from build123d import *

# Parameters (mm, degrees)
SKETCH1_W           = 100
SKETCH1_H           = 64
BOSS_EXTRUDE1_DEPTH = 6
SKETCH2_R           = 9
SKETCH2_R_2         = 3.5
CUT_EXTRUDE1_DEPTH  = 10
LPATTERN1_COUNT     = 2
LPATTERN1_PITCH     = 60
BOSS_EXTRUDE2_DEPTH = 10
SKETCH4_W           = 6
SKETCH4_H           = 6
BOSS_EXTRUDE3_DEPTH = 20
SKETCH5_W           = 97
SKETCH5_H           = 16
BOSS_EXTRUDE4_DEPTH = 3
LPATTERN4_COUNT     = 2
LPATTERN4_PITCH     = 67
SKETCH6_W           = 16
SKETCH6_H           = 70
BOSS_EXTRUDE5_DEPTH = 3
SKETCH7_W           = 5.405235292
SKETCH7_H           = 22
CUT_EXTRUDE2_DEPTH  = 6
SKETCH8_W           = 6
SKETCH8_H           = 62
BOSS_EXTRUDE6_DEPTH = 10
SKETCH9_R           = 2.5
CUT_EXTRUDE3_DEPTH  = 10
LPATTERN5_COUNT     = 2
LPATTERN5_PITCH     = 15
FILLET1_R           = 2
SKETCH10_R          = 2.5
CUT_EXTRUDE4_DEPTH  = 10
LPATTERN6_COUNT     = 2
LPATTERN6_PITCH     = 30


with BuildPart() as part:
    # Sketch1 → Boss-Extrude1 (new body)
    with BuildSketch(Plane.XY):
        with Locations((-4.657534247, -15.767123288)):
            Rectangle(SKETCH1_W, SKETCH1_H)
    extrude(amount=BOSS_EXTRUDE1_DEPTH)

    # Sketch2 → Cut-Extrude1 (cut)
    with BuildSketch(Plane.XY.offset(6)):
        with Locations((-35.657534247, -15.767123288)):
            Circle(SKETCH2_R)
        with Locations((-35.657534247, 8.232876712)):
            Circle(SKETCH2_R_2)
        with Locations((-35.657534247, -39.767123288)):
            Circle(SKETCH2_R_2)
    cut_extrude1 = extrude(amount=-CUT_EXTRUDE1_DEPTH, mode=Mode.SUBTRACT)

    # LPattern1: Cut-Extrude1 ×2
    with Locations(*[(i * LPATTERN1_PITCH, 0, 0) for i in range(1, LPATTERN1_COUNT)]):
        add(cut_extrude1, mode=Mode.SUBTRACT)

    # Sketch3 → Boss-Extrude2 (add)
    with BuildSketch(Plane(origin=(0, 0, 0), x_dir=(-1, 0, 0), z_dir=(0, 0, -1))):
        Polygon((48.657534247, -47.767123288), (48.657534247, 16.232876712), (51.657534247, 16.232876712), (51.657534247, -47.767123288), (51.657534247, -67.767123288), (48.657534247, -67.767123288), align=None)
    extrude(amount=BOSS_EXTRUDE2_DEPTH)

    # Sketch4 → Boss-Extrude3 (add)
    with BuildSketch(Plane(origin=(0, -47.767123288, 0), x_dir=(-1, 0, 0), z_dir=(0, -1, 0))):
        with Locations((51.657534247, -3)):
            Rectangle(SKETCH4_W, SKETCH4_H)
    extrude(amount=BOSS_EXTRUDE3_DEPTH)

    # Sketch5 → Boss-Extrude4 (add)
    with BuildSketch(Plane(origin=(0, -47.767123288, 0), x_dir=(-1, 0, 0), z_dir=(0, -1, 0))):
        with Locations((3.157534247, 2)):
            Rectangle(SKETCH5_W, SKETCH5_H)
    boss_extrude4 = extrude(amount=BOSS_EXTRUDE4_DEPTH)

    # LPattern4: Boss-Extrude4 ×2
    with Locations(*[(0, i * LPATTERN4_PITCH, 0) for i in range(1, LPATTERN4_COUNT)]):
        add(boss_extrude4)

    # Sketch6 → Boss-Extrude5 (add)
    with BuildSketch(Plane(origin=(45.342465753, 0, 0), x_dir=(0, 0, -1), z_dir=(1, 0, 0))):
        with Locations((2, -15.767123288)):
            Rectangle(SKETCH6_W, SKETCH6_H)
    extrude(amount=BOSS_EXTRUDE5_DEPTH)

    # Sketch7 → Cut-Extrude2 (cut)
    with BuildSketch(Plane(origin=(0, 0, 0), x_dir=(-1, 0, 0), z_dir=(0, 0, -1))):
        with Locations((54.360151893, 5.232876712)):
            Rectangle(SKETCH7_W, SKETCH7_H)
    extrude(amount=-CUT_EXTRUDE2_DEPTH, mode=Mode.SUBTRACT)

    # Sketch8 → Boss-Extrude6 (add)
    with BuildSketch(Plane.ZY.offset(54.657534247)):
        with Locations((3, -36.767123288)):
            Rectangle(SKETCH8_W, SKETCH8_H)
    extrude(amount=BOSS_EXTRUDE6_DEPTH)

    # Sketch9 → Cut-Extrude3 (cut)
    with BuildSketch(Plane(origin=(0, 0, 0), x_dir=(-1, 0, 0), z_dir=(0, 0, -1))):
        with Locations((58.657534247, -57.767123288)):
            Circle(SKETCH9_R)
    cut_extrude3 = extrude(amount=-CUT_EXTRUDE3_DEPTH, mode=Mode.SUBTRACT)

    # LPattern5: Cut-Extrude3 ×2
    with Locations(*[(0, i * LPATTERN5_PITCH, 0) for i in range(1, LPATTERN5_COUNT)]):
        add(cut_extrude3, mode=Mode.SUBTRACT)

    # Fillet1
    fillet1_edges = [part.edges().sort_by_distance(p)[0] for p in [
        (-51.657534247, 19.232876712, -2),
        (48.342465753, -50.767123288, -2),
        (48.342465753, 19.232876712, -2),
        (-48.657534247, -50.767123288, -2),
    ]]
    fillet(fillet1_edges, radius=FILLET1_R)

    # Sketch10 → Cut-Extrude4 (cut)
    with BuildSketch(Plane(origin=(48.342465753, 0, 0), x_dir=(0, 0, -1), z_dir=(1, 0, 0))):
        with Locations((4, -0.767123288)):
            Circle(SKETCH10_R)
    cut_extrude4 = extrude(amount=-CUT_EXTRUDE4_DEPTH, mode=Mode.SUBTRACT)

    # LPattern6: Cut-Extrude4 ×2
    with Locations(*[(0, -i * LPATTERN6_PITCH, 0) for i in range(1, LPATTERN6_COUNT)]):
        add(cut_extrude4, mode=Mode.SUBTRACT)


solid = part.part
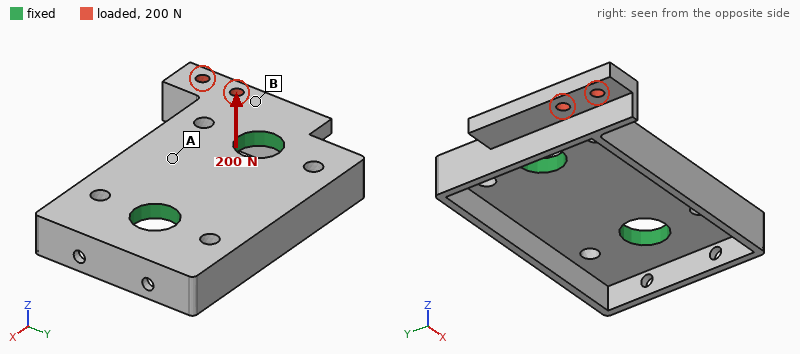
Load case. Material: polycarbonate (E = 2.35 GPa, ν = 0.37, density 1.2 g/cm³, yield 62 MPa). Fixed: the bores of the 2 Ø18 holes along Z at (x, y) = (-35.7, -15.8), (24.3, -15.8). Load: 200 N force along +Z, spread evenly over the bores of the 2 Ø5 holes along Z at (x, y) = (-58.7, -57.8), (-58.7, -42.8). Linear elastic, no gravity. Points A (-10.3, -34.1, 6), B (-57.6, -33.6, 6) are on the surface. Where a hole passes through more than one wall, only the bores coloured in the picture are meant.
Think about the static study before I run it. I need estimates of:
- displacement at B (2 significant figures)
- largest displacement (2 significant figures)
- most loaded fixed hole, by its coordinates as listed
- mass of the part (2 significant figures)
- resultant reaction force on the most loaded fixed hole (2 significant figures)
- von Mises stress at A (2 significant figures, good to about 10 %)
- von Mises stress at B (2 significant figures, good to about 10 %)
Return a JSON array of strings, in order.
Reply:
["0.42 mm", "1.6 mm", "(-35.7, -15.8)", "64 g", "230 N", "2.7 MPa", "6.7 MPa"]
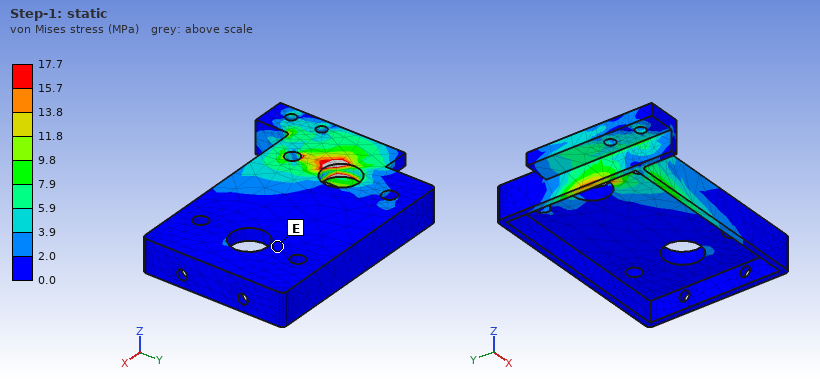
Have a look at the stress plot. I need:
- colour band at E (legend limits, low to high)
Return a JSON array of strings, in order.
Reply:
["0.0 to 2.0 MPa"]
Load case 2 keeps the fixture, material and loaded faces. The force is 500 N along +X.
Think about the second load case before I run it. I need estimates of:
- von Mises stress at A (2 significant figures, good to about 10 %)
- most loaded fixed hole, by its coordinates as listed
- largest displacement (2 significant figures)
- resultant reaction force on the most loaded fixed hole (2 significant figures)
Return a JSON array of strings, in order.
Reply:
["1.8 MPa", "(-35.7, -15.8)", "0.36 mm", "360 N"]
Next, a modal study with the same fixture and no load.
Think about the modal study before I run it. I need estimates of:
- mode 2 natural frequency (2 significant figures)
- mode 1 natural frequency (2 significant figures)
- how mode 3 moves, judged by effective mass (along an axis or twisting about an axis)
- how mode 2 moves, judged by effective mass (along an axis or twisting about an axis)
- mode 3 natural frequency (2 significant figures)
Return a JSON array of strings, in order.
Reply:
["1200 Hz", "970 Hz", "along Z", "twisting about X", "1400 Hz"]
